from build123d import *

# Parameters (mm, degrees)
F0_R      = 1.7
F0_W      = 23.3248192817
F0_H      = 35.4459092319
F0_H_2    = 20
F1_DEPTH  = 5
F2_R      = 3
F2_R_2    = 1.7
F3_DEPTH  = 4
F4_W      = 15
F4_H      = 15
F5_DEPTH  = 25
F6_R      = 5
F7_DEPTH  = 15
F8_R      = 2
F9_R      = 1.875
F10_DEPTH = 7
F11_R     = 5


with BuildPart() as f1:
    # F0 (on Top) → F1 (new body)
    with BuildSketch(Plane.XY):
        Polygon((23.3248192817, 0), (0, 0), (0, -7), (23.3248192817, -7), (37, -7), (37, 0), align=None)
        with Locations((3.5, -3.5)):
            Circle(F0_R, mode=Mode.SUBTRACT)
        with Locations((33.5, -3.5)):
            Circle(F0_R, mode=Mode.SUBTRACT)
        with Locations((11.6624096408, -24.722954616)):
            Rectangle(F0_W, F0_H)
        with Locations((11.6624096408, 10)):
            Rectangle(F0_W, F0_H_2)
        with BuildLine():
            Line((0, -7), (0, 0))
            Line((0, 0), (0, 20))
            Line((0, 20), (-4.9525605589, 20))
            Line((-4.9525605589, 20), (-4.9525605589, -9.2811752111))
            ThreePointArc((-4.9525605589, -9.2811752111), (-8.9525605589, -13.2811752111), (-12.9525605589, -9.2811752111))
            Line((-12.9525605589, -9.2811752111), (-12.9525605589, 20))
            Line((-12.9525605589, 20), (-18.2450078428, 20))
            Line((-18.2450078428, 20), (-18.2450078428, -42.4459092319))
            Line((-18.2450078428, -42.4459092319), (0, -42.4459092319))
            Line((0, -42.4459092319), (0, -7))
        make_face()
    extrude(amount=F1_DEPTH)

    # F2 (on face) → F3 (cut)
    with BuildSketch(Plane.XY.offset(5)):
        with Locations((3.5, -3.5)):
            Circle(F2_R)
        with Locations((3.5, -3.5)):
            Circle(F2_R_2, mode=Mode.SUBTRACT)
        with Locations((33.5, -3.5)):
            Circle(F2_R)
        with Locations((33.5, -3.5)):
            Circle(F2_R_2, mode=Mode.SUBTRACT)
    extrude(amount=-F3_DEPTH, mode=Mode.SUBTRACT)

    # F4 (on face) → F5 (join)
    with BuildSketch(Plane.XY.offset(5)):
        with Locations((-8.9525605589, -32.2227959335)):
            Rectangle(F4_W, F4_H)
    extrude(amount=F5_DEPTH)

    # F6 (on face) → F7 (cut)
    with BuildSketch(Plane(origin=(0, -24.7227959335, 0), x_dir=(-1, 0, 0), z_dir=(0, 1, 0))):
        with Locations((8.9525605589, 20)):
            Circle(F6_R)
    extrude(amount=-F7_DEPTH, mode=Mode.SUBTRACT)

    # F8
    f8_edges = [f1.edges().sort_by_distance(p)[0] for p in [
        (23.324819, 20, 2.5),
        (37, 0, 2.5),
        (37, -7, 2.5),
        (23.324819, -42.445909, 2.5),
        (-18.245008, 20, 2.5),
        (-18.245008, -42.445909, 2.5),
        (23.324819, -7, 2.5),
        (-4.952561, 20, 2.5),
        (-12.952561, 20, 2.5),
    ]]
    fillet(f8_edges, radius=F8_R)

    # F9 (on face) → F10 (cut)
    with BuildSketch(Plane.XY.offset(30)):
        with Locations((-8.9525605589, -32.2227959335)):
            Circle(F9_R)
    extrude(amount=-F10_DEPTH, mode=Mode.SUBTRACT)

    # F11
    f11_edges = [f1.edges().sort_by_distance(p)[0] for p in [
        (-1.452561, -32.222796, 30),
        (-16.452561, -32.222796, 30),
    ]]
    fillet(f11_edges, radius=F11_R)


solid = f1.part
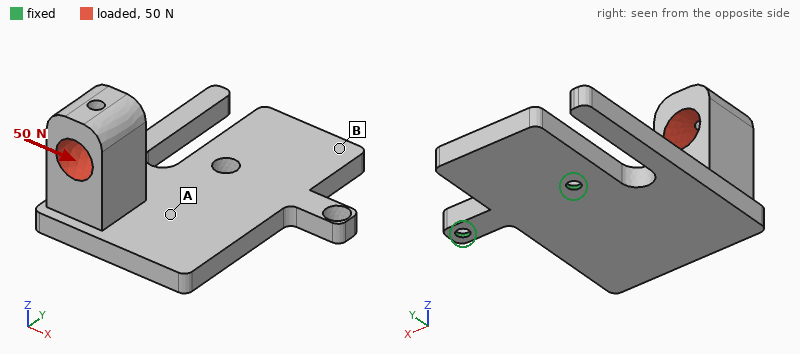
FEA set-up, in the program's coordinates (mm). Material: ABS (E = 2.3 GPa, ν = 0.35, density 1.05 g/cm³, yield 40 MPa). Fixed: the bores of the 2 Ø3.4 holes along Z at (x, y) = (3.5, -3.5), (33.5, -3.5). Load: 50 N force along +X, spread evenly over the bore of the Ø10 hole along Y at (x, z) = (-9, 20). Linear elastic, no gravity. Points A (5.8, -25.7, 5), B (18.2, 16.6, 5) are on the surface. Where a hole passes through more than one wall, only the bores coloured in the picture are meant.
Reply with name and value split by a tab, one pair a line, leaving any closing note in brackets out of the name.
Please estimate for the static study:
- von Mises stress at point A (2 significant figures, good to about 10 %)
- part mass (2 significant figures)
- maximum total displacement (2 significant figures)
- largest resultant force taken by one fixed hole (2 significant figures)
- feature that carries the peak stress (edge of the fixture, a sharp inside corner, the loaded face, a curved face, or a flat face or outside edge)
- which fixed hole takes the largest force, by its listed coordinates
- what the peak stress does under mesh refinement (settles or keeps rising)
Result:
von Mises stress at point A	5.6 MPa
part mass	17 g
maximum total displacement	1.0 mm
largest resultant force taken by one fixed hole	90 N
feature that carries the peak stress	edge of the fixture
which fixed hole takes the largest force, by its listed coordinates	(33.5, -3.5)
what the peak stress does under mesh refinement	keeps rising
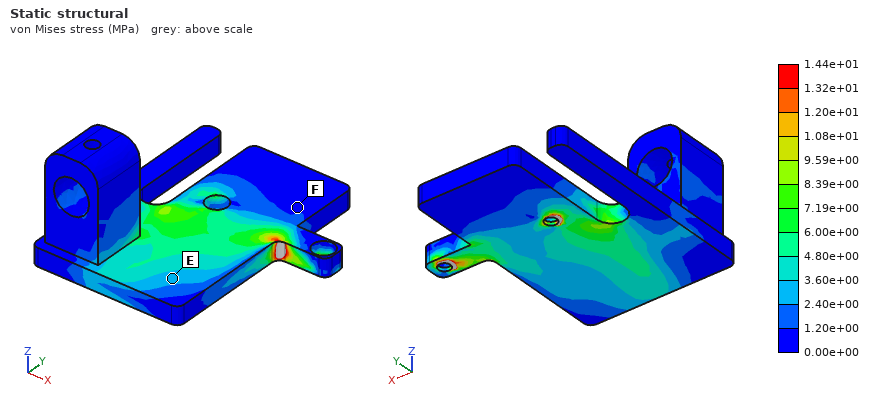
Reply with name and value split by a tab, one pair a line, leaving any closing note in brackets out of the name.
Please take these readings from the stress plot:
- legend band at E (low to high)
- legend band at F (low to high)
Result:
legend band at E	2.40e+00 to 3.60e+00 MPa
legend band at F	0.00e+00 to 1.20e+00 MPa
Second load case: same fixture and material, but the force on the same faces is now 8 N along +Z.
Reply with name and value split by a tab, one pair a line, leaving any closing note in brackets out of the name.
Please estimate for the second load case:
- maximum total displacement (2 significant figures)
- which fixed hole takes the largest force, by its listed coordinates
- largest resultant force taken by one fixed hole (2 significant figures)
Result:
maximum total displacement	0.90 mm
which fixed hole takes the largest force, by its listed coordinates	(3.5, -3.5)
largest resultant force taken by one fixed hole	12 N
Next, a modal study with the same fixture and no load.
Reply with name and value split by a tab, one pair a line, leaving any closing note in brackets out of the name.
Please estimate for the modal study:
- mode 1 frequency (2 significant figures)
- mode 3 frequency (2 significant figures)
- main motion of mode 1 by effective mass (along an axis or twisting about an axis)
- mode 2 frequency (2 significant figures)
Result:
mode 1 frequency	180 Hz
mode 3 frequency	760 Hz
main motion of mode 1 by effective mass	along Z
mode 2 frequency	540 Hz
